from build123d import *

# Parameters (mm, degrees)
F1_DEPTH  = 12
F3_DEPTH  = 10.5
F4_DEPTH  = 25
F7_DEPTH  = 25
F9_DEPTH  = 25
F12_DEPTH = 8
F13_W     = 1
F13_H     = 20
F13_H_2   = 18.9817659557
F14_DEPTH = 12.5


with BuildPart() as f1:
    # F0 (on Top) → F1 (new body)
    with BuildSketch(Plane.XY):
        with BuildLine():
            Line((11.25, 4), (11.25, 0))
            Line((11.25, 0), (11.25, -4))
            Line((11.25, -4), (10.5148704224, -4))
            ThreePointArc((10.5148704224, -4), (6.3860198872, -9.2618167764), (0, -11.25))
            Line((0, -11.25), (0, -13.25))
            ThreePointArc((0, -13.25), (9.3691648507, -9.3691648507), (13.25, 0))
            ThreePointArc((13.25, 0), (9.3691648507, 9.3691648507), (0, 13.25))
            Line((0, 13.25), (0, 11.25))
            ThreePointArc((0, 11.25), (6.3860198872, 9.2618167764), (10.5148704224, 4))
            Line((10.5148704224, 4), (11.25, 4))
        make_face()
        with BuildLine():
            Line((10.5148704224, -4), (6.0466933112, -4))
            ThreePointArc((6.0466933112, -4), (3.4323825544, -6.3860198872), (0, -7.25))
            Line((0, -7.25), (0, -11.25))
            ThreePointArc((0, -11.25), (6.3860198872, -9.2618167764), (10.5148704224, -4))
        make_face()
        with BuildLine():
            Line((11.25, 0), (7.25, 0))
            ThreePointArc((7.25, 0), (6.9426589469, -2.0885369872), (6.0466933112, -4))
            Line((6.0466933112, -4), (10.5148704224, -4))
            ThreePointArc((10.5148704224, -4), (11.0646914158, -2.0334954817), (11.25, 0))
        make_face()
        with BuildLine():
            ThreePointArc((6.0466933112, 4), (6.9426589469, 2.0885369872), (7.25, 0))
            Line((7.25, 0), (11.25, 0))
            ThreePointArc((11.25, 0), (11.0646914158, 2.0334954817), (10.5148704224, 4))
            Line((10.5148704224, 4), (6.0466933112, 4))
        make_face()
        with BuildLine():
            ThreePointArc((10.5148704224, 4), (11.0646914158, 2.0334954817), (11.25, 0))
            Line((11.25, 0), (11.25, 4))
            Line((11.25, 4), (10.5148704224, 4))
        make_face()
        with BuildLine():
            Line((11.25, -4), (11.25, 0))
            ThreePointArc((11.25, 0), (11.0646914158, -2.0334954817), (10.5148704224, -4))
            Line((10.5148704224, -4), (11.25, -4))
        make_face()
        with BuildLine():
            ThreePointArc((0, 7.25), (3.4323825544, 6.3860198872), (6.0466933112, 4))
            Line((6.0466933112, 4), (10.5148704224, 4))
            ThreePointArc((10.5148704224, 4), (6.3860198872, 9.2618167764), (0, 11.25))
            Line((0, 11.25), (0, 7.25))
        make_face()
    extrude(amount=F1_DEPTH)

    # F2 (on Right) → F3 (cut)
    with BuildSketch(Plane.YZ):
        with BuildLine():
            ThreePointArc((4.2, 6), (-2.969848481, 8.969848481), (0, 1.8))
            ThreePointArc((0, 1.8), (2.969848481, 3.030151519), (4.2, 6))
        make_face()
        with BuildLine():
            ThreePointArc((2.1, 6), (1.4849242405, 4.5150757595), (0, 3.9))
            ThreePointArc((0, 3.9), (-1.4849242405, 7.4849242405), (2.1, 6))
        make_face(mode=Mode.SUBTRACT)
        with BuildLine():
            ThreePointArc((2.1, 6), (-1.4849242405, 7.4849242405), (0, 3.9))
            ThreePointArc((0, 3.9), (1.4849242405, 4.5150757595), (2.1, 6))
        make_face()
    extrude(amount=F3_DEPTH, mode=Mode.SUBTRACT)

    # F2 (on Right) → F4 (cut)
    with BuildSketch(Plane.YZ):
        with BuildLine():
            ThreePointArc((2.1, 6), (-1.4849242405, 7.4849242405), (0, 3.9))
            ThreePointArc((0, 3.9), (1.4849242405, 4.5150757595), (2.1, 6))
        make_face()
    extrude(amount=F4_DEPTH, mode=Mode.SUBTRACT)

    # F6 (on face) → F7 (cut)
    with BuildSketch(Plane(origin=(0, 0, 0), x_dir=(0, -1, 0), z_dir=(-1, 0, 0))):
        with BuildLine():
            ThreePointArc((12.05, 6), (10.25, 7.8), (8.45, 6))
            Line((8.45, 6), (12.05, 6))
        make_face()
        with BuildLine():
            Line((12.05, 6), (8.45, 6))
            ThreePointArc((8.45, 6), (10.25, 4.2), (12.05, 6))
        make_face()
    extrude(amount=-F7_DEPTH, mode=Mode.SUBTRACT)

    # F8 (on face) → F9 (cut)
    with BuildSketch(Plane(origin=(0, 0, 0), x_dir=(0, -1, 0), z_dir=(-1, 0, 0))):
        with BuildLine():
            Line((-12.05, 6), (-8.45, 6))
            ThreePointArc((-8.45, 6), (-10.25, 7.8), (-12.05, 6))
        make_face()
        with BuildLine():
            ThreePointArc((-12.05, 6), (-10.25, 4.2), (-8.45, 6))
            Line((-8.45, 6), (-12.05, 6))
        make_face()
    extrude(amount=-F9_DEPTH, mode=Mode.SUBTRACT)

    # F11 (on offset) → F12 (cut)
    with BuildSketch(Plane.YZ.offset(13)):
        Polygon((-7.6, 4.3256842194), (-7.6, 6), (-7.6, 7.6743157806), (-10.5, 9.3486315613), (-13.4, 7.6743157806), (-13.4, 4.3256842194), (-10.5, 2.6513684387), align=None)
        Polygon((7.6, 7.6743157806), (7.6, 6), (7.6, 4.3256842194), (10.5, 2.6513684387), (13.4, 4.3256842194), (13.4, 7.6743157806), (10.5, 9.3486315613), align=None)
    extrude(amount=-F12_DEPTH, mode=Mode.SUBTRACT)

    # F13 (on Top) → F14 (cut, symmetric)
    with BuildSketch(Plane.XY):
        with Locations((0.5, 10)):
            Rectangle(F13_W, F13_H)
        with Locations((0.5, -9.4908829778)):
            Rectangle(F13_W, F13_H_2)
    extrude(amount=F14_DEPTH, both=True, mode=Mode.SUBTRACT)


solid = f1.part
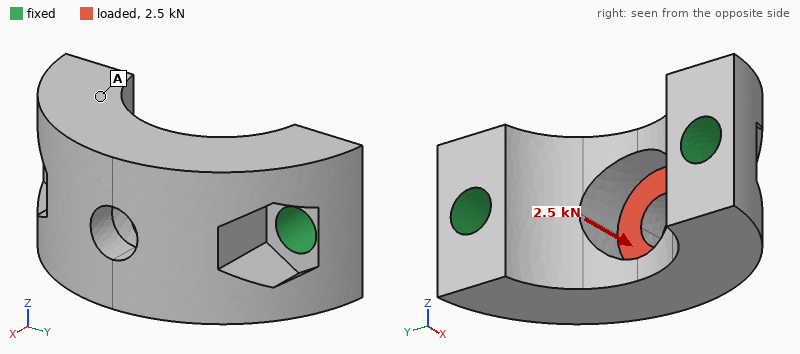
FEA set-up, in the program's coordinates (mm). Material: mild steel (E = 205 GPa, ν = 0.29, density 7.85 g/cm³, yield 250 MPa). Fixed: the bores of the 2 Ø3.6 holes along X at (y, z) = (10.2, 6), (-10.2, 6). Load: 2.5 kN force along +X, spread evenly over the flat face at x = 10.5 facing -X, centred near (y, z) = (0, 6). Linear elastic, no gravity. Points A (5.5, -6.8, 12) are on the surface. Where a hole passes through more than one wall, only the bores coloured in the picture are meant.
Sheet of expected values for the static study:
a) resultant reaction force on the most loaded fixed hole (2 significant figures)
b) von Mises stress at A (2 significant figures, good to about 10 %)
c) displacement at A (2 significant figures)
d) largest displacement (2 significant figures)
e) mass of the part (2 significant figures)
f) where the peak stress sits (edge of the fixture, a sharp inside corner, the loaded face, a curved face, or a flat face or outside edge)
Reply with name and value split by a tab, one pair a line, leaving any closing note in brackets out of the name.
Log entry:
resultant reaction force on the most loaded fixed hole	1.5 kN
von Mises stress at A	19 MPa
displacement at A	1.7 µm
largest displacement	6.8 µm
mass of the part	13 g
where the peak stress sits	a curved face
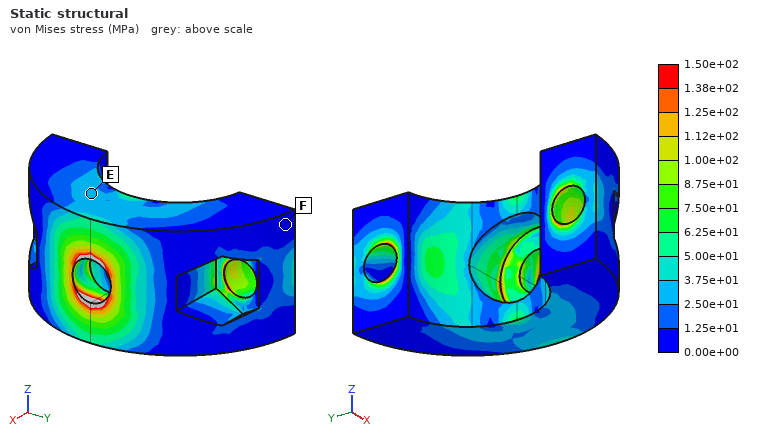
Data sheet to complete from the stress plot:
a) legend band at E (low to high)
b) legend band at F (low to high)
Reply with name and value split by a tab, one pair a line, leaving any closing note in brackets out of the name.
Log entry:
legend band at E	2.50e+01 to 3.75e+01 MPa
legend band at F	0.00e+00 to 1.25e+01 MPa
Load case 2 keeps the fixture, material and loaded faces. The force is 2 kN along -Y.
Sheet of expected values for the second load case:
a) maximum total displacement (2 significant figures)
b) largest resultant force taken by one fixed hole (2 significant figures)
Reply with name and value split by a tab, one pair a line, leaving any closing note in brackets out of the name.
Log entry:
maximum total displacement	5.6 µm
largest resultant force taken by one fixed hole	1.2 kN
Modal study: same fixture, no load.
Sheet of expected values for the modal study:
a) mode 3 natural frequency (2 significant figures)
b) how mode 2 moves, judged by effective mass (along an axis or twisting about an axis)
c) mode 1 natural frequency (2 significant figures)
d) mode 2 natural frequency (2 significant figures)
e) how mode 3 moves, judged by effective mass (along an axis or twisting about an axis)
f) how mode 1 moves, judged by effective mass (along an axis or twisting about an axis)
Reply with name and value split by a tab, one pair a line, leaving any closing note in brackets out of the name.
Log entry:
mode 3 natural frequency	49 kHz
how mode 2 moves, judged by effective mass	along Y
mode 1 natural frequency	24 kHz
mode 2 natural frequency	44 kHz
how mode 3 moves, judged by effective mass	twisting about X
how mode 1 moves, judged by effective mass	along Z
